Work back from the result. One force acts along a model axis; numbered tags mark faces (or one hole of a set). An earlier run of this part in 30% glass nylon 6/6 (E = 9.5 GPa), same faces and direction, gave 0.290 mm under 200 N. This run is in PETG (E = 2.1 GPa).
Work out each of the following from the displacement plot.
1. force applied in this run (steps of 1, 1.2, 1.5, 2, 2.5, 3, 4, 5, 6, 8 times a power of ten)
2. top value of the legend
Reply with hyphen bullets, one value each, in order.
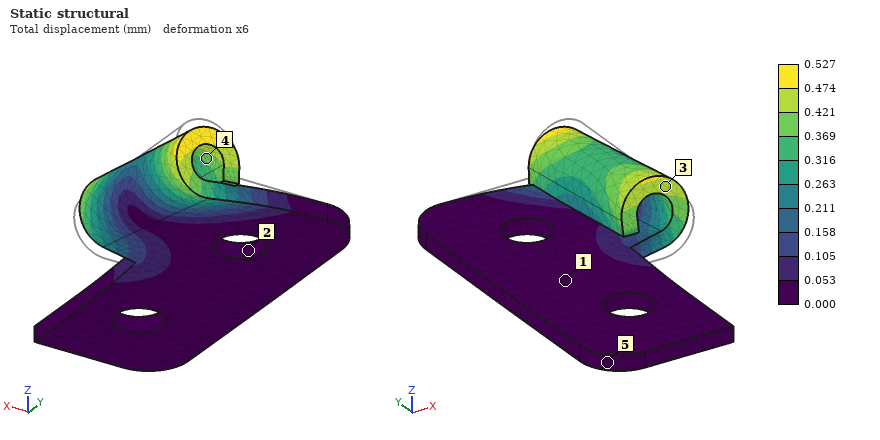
- 80 N
- 0.527 mm
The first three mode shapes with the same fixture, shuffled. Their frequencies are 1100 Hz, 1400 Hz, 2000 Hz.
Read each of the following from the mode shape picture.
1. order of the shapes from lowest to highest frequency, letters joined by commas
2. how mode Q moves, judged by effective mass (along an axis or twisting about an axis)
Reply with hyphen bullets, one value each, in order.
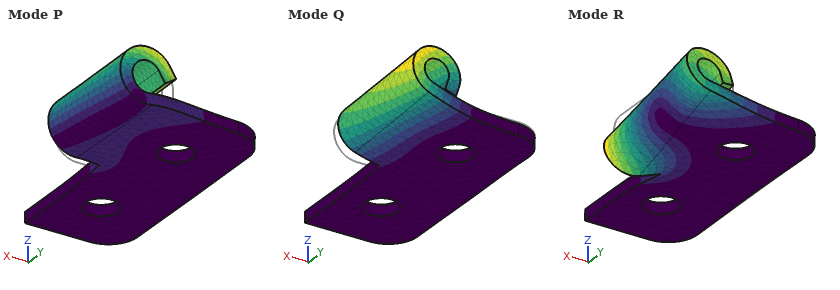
- Q, R, P
- along Z
